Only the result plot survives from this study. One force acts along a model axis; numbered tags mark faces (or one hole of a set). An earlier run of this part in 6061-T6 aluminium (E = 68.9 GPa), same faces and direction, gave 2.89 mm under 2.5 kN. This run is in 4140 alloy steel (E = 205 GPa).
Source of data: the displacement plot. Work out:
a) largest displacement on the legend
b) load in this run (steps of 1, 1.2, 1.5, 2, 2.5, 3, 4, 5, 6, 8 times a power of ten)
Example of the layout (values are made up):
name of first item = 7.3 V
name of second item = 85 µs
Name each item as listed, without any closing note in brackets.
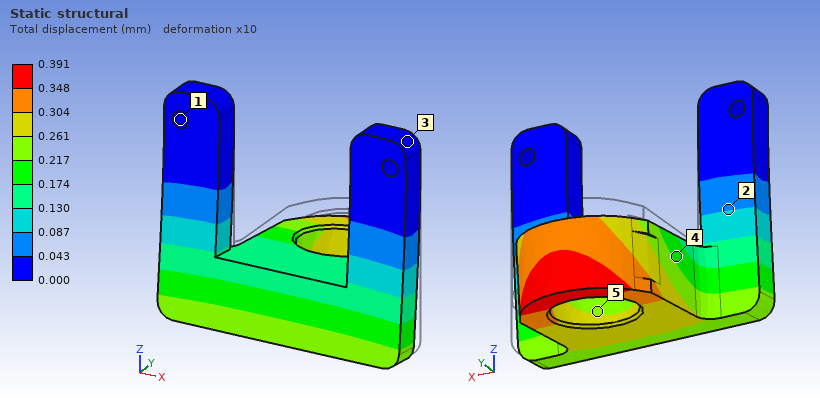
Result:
largest displacement on the legend = 0.391 mm
load in this run = 1 kN
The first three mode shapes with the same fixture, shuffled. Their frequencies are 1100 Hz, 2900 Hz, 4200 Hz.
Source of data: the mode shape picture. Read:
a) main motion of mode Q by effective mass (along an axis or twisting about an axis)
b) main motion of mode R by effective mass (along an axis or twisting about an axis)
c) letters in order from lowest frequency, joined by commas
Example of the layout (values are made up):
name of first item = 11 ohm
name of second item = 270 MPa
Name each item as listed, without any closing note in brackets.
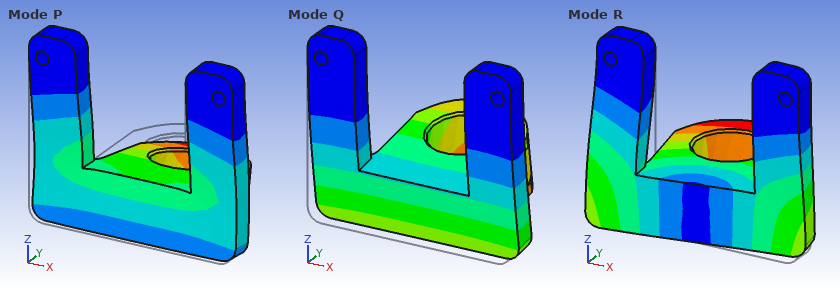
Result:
main motion of mode Q by effective mass = along Y
main motion of mode R by effective mass = along X
letters in order from lowest frequency, joined by commas = Q, R, P
